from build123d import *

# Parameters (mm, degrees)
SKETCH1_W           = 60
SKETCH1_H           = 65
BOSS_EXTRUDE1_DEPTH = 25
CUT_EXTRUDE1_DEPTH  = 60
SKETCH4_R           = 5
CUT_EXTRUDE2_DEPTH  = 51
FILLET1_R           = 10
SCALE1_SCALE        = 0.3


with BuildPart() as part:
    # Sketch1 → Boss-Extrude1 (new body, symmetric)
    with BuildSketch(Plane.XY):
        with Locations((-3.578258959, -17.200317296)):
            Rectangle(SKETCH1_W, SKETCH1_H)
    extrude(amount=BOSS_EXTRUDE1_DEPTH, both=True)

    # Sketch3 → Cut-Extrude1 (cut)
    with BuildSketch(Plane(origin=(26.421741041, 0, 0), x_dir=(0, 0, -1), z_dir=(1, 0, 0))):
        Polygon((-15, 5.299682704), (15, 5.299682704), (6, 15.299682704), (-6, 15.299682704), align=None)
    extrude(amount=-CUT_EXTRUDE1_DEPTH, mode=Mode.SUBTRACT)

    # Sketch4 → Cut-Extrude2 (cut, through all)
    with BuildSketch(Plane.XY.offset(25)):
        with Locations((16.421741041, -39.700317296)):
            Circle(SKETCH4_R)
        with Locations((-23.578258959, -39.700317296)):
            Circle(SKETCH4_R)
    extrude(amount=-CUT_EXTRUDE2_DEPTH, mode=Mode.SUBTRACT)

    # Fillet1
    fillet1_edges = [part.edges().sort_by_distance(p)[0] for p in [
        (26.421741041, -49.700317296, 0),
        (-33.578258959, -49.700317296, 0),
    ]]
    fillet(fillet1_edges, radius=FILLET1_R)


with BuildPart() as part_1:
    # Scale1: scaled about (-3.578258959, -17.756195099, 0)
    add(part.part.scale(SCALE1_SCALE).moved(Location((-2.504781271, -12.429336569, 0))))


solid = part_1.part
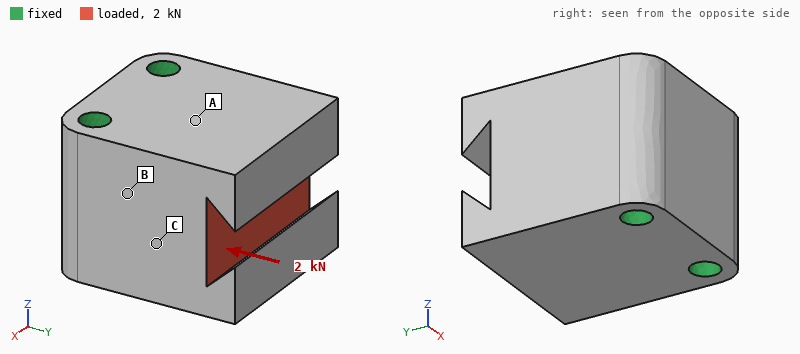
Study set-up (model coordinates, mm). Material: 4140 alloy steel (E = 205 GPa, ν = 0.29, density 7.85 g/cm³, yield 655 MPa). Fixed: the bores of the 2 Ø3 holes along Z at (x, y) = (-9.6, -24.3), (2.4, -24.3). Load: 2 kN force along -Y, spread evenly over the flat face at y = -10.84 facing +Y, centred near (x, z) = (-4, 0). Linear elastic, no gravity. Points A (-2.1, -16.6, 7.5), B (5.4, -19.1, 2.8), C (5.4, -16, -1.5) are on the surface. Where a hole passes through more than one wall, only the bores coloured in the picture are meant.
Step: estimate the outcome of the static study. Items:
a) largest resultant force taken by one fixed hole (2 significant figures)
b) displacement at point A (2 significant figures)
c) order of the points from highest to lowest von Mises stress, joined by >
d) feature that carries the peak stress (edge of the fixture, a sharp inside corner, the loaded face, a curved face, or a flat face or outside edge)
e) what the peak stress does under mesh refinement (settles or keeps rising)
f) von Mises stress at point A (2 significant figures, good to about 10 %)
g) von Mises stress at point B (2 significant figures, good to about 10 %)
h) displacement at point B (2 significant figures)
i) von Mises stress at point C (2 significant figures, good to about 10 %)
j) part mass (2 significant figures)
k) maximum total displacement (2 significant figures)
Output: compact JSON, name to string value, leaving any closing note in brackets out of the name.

{"largest resultant force taken by one fixed hole": "1.0 kN", "displacement at point A": "0.28 µm", "order of the points from highest to lowest von Mises stress, joined by >": "C > B > A", "feature that carries the peak stress": "edge of the fixture", "what the peak stress does under mesh refinement": "keeps rising", "von Mises stress at point A": "2.4 MPa", "von Mises stress at point B": "9.1 MPa", "displacement at point B": "0.22 µm", "von Mises stress at point C": "12 MPa", "part mass": "37 g", "maximum total displacement": "0.72 µm"}
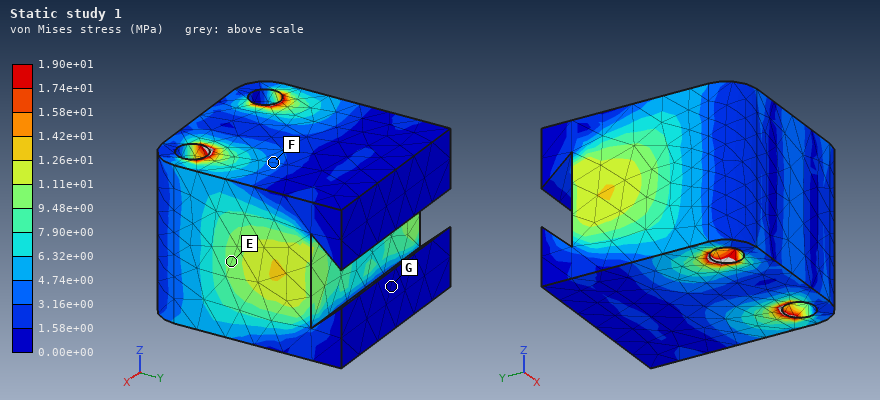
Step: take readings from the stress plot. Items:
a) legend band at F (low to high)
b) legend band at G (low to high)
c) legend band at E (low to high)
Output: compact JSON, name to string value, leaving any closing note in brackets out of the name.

{"legend band at F": "3.16e+00 to 4.74e+00 MPa", "legend band at G": "0.00e+00 to 1.58e+00 MPa", "legend band at E": "9.48e+00 to 1.11e+01 MPa"}
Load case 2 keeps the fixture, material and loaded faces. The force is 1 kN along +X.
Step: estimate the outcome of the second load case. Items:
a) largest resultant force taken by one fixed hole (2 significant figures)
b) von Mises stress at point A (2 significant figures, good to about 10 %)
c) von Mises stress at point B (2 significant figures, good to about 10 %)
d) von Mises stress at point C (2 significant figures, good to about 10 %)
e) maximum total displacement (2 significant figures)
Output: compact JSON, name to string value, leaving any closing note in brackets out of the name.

{"largest resultant force taken by one fixed hole": "1.1 kN", "von Mises stress at point A": "9.4 MPa", "von Mises stress at point B": "9.7 MPa", "von Mises stress at point C": "8.8 MPa", "maximum total displacement": "1.6 µm"}
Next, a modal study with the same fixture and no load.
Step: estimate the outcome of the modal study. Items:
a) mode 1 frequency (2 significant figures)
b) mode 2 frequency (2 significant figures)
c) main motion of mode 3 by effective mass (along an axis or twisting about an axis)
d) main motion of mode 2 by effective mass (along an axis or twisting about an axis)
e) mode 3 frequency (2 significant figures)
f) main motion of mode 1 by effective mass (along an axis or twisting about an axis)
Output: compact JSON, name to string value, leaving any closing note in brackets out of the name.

{"mode 1 frequency": "32 kHz", "mode 2 frequency": "38 kHz", "main motion of mode 3 by effective mass": "twisting about Y", "main motion of mode 2 by effective mass": "along X", "mode 3 frequency": "48 kHz", "main motion of mode 1 by effective mass": "along Z"}
